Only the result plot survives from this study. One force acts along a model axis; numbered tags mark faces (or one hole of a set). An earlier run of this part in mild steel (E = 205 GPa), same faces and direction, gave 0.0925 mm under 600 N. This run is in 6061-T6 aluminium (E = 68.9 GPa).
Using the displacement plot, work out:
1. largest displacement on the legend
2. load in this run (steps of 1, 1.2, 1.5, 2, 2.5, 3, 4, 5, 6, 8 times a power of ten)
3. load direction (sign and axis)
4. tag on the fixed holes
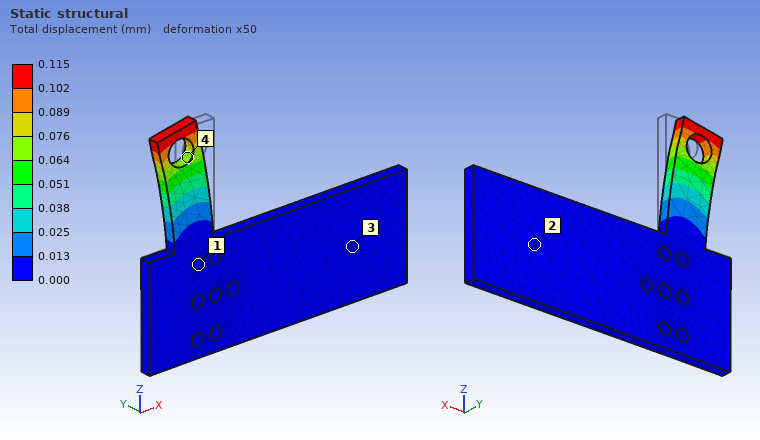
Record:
0.115 mm
250 N
-X
1
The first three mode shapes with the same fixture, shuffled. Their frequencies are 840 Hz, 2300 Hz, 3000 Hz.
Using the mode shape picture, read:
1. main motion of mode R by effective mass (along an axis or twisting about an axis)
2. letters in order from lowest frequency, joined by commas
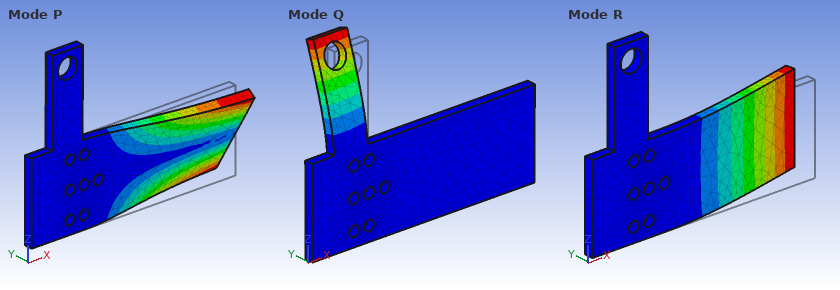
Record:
along Y
R, Q, P
